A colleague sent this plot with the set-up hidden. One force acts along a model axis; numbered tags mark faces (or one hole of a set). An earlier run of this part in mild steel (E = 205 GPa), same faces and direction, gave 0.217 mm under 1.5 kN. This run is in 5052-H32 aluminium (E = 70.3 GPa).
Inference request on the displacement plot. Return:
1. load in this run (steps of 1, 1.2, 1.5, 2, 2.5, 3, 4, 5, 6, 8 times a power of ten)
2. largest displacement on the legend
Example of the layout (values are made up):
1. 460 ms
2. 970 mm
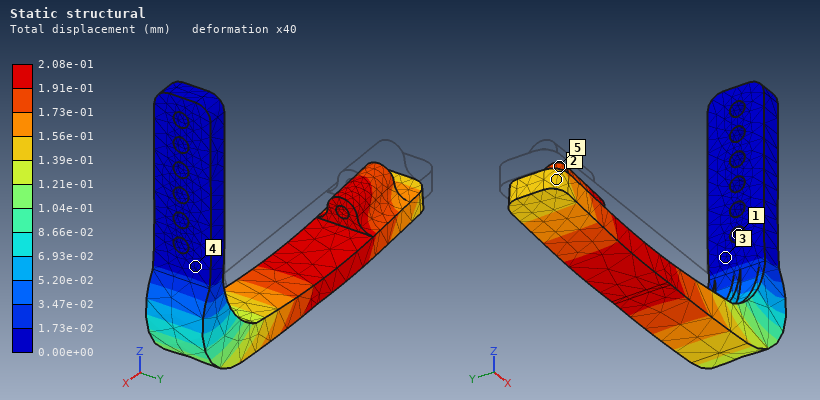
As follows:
1. 500 N
2. 2.08e-01 mm
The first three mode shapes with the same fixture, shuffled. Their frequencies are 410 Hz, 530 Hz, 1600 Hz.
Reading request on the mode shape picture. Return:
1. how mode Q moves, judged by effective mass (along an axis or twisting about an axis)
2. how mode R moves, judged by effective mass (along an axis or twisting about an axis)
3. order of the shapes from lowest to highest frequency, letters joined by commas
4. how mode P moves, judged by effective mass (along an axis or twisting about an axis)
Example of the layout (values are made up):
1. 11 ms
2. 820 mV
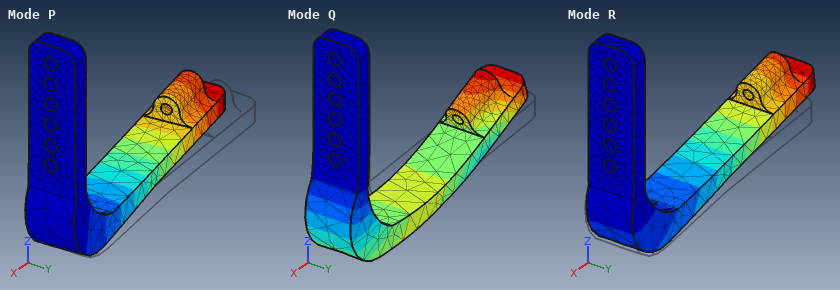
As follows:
1. along X
2. along Z
3. R, P, Q
4. along Y
